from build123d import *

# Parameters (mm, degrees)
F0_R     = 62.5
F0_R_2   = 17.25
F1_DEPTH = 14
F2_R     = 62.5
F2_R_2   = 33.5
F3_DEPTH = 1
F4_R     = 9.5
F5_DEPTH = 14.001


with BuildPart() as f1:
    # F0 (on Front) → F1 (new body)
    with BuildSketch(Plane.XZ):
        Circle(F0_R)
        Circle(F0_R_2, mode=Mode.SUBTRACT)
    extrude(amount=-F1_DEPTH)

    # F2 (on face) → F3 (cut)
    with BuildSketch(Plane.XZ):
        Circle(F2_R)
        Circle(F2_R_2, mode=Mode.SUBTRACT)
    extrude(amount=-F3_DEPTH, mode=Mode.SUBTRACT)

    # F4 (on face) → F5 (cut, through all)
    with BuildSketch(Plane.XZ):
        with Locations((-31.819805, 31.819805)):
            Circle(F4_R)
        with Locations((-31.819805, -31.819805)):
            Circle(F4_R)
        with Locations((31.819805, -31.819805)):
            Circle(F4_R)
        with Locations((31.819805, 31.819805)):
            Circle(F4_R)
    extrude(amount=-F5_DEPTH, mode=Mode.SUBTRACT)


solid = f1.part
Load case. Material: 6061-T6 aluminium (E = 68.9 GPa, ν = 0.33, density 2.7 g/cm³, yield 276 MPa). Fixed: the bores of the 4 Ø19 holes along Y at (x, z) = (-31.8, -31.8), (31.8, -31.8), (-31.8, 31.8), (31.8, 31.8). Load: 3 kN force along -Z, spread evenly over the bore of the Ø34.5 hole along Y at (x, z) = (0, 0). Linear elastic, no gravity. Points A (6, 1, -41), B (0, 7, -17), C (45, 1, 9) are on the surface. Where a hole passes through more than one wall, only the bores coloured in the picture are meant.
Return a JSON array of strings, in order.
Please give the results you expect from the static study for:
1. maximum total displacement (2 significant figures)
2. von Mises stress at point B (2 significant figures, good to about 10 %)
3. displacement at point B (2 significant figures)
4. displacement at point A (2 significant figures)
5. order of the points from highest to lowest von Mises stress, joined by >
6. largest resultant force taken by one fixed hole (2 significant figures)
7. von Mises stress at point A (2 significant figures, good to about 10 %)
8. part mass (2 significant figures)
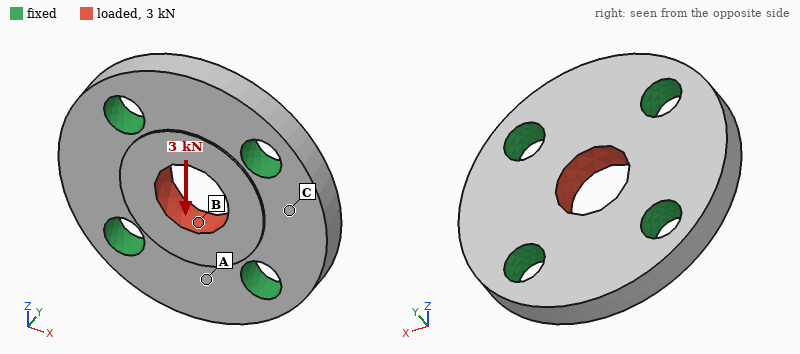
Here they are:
["1.1 µm", "1.8 MPa", "1.00 µm", "0.56 µm", "B > A > C", "780 N", "0.91 MPa", "370 g"]
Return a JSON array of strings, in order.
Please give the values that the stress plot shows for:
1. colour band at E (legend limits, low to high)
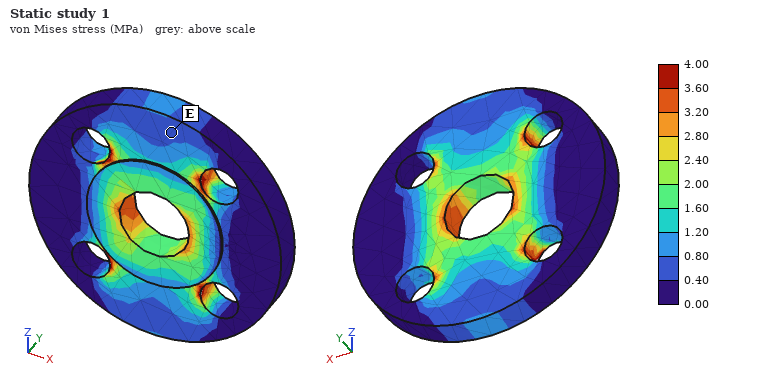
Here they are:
["0.40 to 0.80 MPa"]
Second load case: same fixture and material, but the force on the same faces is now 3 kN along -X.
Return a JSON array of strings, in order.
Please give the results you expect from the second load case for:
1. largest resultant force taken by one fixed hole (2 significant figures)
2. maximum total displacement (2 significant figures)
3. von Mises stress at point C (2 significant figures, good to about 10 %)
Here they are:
["780 N", "1.1 µm", "0.87 MPa"]
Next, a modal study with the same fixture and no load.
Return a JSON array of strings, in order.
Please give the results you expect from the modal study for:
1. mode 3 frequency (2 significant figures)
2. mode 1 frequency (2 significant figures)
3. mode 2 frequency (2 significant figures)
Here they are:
["13 kHz", "13 kHz", "13 kHz"]
